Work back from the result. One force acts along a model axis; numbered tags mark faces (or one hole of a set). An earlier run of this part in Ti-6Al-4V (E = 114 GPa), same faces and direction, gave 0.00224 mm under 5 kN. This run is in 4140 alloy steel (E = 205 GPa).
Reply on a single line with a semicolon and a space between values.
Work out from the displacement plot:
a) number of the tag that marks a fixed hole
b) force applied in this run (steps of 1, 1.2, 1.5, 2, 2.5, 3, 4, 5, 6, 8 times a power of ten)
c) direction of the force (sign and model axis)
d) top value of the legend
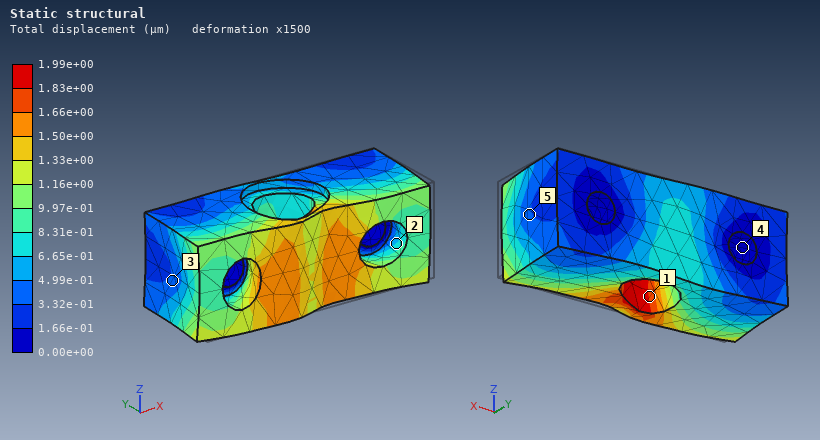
4; 8 kN; -X; 1.99e+00 µm
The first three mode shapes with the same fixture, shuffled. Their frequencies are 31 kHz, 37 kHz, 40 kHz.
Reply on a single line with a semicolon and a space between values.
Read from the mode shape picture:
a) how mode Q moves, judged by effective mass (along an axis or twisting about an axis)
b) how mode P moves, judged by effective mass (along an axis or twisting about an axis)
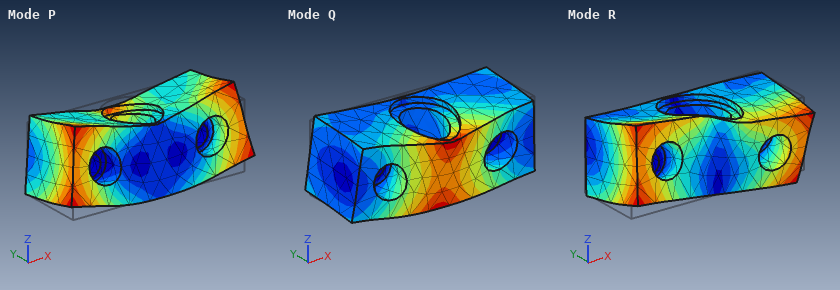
along Z; twisting about X
